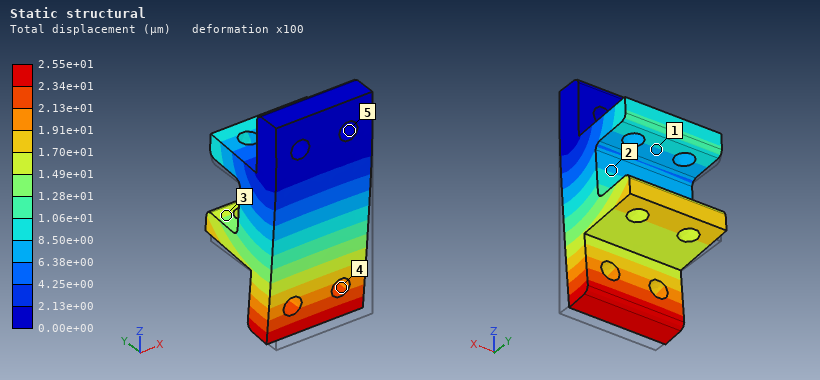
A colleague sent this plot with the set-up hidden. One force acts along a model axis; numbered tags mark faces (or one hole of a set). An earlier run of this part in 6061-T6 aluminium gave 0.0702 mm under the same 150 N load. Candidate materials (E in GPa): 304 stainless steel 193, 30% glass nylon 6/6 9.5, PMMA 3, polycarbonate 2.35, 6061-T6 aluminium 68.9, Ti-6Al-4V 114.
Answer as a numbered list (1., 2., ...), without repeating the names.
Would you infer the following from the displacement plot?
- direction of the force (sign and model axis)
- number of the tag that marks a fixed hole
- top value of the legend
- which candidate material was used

1. +Y
2. 5
3. 2.55e+01 µm
4. 304 stainless steel
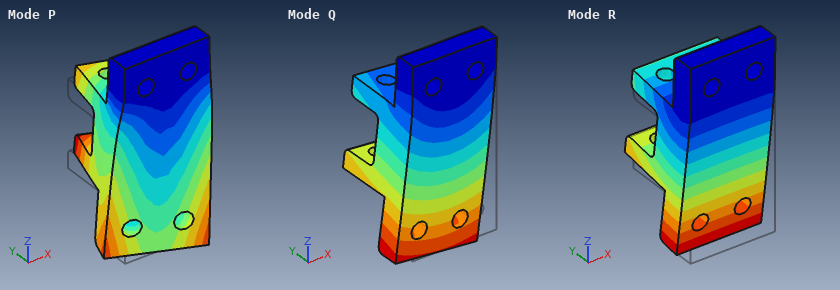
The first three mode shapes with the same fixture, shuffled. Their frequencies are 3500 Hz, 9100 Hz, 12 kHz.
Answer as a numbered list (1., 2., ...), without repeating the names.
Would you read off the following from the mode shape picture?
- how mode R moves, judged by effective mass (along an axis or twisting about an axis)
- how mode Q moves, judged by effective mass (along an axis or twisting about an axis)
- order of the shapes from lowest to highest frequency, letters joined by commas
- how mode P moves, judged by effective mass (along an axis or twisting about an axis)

1. along Y
2. along X
3. R, Q, P
4. twisting about Z
